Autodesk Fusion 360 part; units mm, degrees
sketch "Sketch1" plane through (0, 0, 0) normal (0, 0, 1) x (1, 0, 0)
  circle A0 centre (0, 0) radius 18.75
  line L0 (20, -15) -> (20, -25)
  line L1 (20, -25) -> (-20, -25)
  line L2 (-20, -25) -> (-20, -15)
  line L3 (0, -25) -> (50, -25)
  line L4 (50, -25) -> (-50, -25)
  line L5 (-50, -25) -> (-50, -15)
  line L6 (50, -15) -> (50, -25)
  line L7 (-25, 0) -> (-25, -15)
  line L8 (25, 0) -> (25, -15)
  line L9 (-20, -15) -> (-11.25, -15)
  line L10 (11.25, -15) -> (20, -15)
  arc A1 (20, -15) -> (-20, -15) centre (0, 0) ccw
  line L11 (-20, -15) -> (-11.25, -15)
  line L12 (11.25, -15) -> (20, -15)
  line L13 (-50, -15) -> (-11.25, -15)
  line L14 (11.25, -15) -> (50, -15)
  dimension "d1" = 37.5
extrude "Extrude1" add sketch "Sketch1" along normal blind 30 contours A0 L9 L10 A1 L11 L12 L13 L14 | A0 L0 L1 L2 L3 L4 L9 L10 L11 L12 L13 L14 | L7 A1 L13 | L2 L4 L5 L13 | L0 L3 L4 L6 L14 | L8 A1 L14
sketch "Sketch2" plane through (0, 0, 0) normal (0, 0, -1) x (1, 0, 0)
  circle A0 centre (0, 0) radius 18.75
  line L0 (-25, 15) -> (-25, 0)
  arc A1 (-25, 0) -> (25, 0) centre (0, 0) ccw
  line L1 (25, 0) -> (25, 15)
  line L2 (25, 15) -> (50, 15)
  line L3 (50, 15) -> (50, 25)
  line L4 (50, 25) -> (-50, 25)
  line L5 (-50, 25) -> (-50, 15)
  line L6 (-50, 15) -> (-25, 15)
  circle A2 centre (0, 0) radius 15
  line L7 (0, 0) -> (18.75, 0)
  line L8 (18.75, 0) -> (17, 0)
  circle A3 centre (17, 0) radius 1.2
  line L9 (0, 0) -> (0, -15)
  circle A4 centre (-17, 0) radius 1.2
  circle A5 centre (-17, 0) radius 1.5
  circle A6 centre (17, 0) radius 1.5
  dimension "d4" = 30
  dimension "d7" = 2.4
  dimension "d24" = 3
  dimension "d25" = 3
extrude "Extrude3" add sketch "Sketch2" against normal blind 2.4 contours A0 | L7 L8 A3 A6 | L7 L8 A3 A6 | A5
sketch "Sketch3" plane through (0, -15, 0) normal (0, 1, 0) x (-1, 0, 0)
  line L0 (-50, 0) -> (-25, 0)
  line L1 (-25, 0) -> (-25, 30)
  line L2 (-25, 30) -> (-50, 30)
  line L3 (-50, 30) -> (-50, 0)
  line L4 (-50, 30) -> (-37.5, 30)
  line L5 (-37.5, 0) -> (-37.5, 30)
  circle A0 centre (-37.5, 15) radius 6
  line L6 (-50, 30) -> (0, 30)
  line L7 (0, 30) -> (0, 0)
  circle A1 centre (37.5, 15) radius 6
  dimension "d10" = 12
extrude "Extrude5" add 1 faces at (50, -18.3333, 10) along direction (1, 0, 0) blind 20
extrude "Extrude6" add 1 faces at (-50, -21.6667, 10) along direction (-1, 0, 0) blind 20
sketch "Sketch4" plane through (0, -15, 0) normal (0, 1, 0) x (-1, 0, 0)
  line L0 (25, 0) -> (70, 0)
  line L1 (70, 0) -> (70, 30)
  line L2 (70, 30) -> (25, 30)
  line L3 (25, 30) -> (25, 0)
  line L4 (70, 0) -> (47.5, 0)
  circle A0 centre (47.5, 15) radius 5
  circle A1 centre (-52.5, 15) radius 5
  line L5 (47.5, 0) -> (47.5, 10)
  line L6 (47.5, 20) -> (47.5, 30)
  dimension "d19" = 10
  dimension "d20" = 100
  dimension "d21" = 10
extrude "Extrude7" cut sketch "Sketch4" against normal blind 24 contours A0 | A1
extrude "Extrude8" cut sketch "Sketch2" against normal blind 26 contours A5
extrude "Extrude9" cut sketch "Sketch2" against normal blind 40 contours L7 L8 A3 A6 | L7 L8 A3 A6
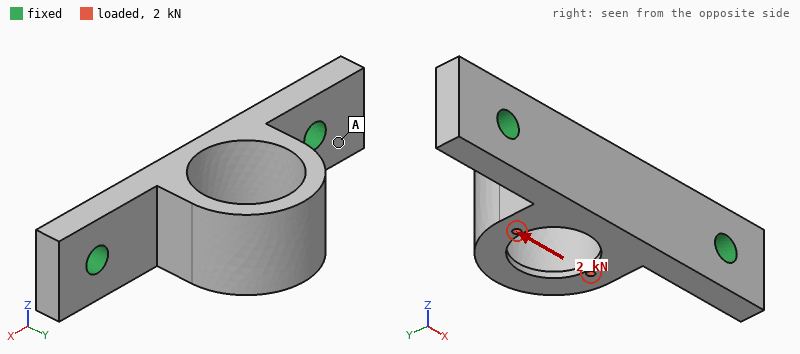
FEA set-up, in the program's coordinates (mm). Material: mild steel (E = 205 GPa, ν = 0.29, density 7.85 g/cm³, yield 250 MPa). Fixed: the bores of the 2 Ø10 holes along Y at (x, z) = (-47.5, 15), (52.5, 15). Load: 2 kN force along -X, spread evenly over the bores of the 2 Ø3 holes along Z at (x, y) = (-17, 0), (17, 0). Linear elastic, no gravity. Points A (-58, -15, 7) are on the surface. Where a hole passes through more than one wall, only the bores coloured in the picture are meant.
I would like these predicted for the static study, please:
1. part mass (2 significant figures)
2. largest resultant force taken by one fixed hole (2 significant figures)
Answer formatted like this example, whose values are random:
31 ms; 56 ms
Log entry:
470 g; 1.2 kN
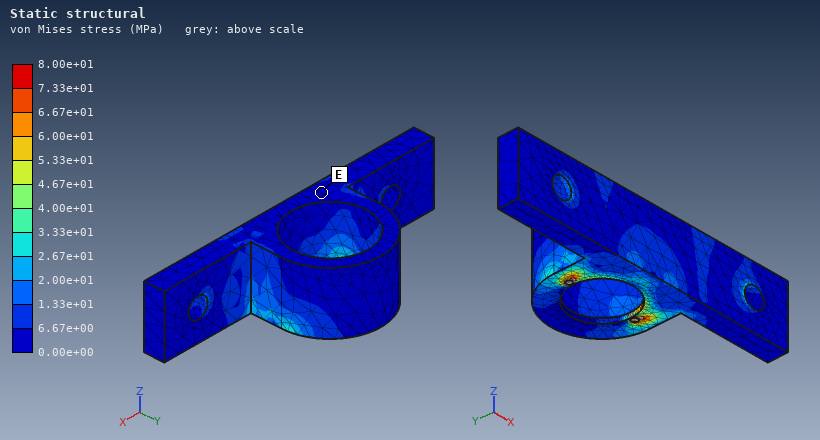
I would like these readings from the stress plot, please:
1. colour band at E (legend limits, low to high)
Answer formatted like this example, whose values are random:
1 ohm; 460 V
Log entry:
0.00e+00 to 6.67e+00 MPa
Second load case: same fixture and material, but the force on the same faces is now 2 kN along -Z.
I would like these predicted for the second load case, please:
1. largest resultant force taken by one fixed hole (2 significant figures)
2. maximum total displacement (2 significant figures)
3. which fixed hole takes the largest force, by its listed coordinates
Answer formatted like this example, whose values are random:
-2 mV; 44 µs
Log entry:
1.1 kN; 37 µm; (-47.5, 15)
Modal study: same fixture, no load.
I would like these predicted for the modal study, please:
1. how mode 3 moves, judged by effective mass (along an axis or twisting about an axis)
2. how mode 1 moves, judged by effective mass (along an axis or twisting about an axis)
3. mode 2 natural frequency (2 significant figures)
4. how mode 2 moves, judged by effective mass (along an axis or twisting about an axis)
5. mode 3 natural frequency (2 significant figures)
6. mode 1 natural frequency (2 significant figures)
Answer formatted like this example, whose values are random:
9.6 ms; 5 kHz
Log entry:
along X; along Z; 4600 Hz; along Y; 5500 Hz; 2900 Hz
